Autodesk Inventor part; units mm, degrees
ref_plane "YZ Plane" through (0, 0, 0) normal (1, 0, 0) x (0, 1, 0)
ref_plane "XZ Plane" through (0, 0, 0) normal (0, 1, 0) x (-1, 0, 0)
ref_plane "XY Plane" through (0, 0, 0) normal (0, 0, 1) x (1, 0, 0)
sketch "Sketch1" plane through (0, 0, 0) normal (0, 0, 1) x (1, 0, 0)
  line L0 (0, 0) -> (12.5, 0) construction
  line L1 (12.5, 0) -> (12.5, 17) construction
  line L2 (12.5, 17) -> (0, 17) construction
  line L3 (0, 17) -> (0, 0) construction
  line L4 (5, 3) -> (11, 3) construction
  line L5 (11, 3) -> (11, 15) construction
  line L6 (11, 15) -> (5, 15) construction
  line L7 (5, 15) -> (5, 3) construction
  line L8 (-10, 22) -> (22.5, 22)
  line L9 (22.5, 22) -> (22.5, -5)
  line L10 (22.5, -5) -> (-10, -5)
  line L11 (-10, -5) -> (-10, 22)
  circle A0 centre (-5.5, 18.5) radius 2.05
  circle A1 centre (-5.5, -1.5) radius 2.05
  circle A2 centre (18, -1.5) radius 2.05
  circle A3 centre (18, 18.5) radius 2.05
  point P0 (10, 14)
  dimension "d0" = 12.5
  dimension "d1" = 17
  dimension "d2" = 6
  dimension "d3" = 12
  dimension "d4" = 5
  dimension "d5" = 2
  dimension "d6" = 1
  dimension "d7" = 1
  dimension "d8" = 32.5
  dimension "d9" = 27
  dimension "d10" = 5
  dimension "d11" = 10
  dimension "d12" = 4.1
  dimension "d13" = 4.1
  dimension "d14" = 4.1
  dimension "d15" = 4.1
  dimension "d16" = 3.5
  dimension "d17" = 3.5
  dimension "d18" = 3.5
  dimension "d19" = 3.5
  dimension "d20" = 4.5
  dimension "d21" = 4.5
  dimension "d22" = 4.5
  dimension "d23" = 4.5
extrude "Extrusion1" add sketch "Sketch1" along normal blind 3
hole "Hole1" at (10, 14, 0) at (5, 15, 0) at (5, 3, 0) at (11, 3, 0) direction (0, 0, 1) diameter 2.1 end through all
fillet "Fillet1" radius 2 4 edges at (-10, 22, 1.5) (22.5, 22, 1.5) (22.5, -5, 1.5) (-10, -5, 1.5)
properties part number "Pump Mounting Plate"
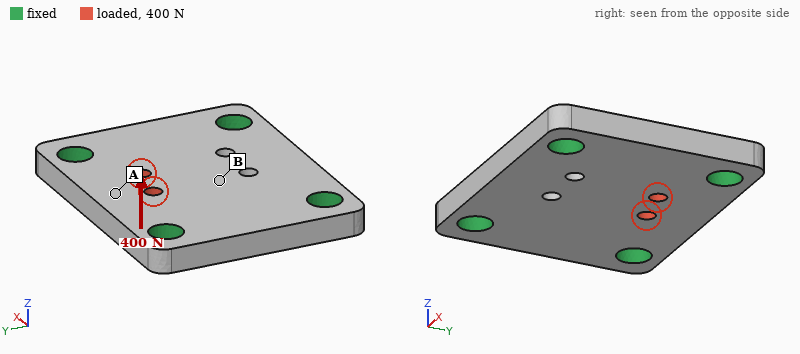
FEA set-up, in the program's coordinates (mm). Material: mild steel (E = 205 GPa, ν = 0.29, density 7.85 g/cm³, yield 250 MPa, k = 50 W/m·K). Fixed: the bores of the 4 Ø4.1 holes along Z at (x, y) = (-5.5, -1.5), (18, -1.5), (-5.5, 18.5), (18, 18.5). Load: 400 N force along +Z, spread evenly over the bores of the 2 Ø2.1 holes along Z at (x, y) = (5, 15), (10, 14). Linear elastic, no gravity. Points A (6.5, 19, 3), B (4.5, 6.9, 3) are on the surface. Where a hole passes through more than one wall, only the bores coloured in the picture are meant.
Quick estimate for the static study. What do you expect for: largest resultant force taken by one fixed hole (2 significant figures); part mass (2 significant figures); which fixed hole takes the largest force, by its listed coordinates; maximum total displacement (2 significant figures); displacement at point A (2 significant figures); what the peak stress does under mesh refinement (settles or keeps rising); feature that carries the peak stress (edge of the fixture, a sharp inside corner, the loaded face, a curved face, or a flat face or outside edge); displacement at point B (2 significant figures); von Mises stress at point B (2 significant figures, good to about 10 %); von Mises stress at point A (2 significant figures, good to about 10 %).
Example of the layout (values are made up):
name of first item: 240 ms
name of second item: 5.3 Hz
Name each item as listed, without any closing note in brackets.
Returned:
largest resultant force taken by one fixed hole: 190 N
part mass: 19 g
which fixed hole takes the largest force, by its listed coordinates: (18, 18.5)
maximum total displacement: 4.2 µm
displacement at point A: 2.9 µm
what the peak stress does under mesh refinement: keeps rising
feature that carries the peak stress: edge of the fixture
displacement at point B: 2.2 µm
von Mises stress at point B: 14 MPa
von Mises stress at point A: 30 MPa
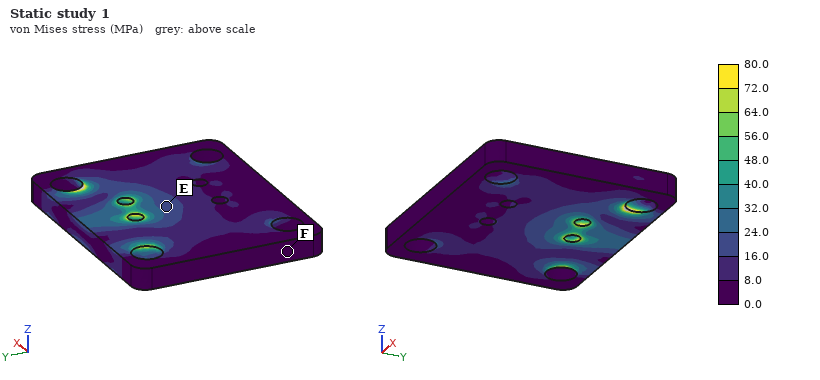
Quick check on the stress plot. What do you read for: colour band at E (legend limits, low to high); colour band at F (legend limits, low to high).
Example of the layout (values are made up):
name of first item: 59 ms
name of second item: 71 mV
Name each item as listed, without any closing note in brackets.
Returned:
colour band at E: 16.0 to 24.0 MPa
colour band at F: 0.0 to 8.0 MPa
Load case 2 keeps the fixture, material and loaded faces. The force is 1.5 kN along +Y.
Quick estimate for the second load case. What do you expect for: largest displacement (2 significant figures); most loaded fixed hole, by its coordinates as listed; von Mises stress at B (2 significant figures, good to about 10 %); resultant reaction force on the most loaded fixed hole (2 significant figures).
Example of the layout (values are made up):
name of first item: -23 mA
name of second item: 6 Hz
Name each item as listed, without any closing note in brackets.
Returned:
largest displacement: 2.2 µm
most loaded fixed hole, by its coordinates as listed: (18, 18.5)
von Mises stress at B: 17 MPa
resultant reaction force on the most loaded fixed hole: 520 N
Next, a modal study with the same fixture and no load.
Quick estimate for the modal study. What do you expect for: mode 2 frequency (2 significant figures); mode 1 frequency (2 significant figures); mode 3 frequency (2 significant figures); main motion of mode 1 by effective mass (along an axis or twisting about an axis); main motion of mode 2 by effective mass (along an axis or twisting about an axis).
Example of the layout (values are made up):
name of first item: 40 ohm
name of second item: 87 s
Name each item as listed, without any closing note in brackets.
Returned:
mode 2 frequency: 36 kHz
mode 1 frequency: 26 kHz
mode 3 frequency: 41 kHz
main motion of mode 1 by effective mass: along Z
main motion of mode 2 by effective mass: twisting about X
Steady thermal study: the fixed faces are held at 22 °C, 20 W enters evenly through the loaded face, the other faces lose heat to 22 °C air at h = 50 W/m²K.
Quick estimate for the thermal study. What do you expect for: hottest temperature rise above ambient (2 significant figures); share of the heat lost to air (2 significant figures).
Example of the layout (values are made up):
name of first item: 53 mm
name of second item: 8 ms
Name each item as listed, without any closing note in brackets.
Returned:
hottest temperature rise above ambient: 51 K
share of the heat lost to air: 5.4 %
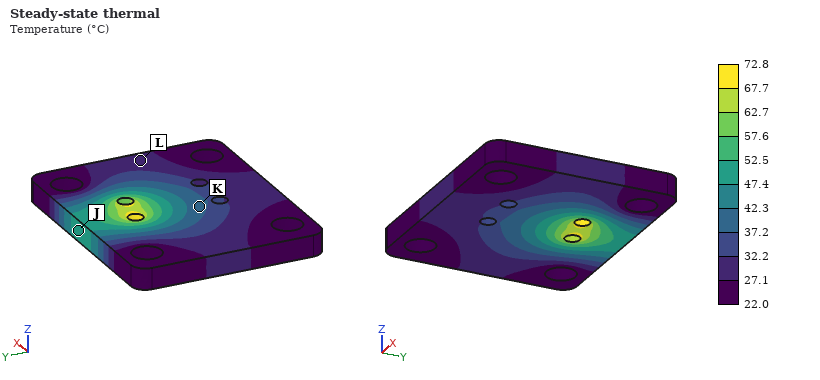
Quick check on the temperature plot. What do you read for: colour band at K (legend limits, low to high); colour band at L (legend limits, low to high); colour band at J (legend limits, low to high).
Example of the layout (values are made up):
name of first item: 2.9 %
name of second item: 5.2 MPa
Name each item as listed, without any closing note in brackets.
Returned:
colour band at K: 37.2 to 42.3 °C
colour band at L: 27.1 to 32.2 °C
colour band at J: 47.4 to 52.5 °C
